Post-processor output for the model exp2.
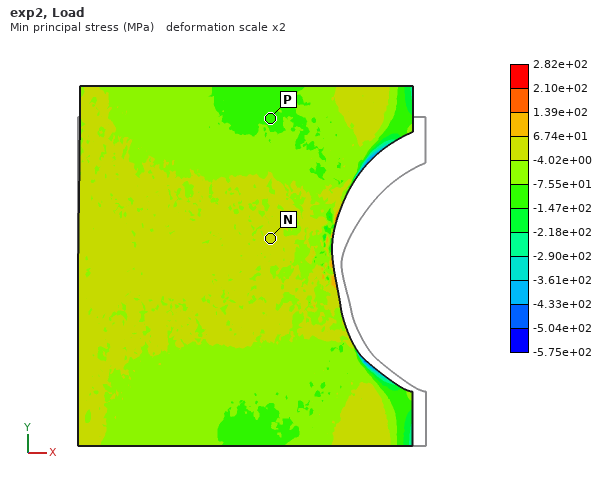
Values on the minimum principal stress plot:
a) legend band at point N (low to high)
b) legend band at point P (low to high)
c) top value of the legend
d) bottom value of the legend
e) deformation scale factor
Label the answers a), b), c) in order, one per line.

a) -4.02e+00 to 6.74e+01 MPa
b) -1.47e+02 to -7.55e+01 MPa
c) 2.82e+02 MPa
d) -5.75e+02 MPa
e) 2
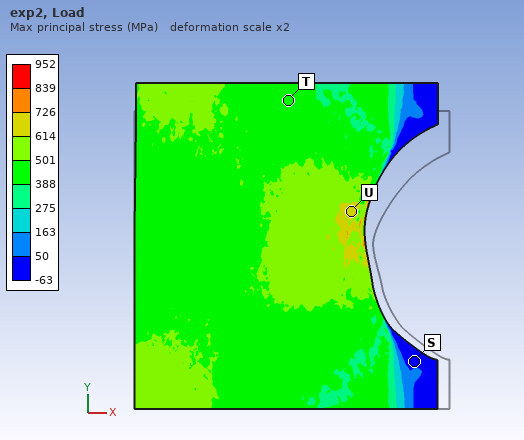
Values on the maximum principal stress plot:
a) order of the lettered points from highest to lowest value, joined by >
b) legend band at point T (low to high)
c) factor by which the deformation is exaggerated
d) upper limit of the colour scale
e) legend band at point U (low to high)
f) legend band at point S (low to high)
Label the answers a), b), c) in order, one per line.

a) U > T > S
b) 388 to 501 MPa
c) 2
d) 952 MPa
e) 614 to 726 MPa
f) -63 to 50 MPa
